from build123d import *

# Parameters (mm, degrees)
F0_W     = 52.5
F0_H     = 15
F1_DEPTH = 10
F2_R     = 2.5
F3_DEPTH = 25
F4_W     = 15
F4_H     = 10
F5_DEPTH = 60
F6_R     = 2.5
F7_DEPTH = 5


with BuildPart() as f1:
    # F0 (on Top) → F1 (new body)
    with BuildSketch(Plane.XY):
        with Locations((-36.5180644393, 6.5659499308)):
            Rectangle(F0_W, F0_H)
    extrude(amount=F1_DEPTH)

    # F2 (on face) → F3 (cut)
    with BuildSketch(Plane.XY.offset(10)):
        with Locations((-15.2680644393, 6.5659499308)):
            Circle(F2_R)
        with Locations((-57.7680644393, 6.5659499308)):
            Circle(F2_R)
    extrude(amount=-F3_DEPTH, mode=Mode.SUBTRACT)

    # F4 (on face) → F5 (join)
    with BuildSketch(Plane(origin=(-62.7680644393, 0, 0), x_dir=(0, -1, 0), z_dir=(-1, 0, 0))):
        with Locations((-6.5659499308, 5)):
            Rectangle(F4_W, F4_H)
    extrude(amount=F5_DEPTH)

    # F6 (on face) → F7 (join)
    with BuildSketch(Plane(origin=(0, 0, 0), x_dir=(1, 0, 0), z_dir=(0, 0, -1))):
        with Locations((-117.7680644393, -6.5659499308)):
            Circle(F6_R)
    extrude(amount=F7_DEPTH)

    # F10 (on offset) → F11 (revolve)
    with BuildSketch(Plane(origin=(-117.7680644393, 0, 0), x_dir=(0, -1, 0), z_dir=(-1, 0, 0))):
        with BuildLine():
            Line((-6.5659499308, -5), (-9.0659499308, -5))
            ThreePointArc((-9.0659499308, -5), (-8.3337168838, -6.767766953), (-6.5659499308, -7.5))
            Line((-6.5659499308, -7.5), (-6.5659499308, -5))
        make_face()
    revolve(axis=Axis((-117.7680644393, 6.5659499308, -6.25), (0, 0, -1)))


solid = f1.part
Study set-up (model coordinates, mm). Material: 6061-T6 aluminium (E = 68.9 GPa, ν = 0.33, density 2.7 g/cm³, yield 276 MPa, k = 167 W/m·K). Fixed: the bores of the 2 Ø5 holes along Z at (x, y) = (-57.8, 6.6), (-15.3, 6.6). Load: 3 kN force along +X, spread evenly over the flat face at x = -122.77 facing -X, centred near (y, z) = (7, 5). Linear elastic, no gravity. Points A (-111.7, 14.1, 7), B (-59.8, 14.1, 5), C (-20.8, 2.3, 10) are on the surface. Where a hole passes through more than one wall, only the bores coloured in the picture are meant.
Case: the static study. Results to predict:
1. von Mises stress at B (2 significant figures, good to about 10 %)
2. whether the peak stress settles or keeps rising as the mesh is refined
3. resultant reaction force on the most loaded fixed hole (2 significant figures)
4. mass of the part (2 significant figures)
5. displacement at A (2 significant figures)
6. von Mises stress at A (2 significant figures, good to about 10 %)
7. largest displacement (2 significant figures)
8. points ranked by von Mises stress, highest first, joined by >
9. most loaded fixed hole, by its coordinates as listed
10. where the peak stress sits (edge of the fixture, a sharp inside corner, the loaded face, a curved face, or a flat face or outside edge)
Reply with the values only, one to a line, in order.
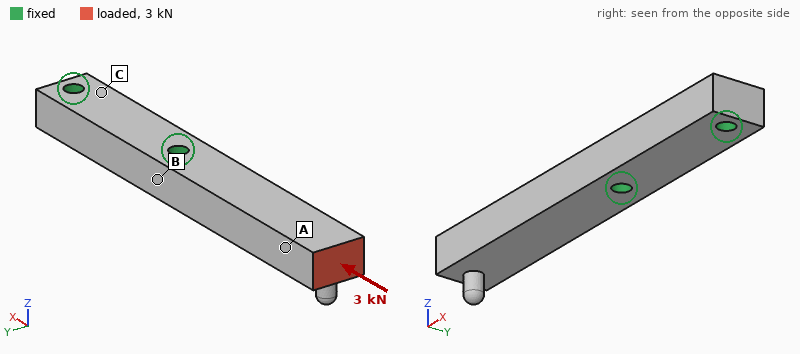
10 MPa
keeps rising
2.9 kN
45 g
16 µm
20 MPa
19 µm
A > B > C
(-57.8, 6.6)
edge of the fixture
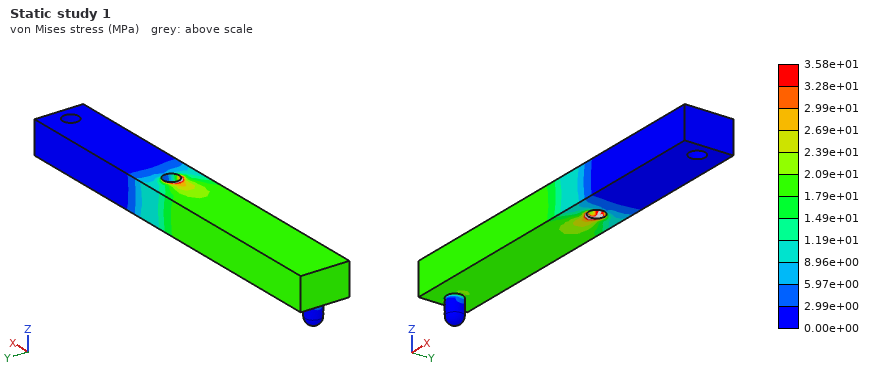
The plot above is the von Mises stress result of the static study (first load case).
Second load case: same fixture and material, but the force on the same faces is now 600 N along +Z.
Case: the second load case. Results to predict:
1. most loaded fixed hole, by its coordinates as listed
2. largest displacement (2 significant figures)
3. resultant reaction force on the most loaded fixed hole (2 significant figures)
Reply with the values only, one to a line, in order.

(-57.8, 6.6)
0.64 mm
690 N
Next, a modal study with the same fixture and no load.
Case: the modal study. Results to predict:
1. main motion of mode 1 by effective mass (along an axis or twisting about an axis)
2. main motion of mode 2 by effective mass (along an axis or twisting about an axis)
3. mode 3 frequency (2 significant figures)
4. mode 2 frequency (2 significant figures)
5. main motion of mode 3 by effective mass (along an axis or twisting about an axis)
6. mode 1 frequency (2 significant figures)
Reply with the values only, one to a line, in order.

along Z
along Y
9900 Hz
2400 Hz
twisting about X
1900 Hz
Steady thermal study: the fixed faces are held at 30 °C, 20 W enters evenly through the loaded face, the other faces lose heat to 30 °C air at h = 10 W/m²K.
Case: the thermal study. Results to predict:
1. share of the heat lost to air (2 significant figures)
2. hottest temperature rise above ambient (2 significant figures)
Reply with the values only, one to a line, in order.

4.2 %
50 K
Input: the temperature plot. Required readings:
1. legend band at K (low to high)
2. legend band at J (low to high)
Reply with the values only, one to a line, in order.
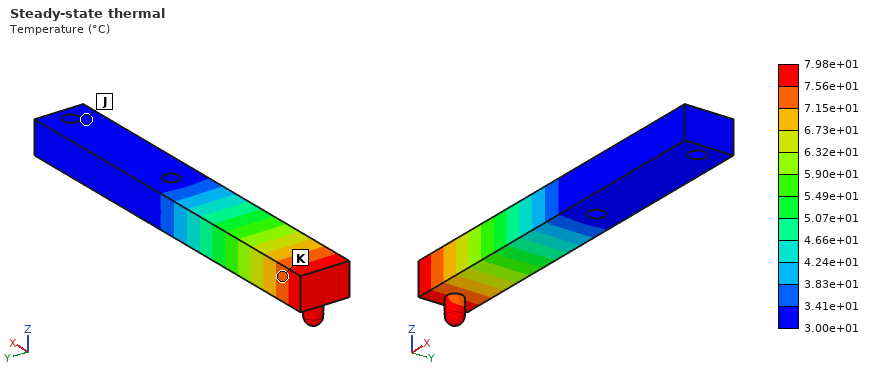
7.15e+01 to 7.56e+01 °C
3.00e+01 to 3.41e+01 °C
